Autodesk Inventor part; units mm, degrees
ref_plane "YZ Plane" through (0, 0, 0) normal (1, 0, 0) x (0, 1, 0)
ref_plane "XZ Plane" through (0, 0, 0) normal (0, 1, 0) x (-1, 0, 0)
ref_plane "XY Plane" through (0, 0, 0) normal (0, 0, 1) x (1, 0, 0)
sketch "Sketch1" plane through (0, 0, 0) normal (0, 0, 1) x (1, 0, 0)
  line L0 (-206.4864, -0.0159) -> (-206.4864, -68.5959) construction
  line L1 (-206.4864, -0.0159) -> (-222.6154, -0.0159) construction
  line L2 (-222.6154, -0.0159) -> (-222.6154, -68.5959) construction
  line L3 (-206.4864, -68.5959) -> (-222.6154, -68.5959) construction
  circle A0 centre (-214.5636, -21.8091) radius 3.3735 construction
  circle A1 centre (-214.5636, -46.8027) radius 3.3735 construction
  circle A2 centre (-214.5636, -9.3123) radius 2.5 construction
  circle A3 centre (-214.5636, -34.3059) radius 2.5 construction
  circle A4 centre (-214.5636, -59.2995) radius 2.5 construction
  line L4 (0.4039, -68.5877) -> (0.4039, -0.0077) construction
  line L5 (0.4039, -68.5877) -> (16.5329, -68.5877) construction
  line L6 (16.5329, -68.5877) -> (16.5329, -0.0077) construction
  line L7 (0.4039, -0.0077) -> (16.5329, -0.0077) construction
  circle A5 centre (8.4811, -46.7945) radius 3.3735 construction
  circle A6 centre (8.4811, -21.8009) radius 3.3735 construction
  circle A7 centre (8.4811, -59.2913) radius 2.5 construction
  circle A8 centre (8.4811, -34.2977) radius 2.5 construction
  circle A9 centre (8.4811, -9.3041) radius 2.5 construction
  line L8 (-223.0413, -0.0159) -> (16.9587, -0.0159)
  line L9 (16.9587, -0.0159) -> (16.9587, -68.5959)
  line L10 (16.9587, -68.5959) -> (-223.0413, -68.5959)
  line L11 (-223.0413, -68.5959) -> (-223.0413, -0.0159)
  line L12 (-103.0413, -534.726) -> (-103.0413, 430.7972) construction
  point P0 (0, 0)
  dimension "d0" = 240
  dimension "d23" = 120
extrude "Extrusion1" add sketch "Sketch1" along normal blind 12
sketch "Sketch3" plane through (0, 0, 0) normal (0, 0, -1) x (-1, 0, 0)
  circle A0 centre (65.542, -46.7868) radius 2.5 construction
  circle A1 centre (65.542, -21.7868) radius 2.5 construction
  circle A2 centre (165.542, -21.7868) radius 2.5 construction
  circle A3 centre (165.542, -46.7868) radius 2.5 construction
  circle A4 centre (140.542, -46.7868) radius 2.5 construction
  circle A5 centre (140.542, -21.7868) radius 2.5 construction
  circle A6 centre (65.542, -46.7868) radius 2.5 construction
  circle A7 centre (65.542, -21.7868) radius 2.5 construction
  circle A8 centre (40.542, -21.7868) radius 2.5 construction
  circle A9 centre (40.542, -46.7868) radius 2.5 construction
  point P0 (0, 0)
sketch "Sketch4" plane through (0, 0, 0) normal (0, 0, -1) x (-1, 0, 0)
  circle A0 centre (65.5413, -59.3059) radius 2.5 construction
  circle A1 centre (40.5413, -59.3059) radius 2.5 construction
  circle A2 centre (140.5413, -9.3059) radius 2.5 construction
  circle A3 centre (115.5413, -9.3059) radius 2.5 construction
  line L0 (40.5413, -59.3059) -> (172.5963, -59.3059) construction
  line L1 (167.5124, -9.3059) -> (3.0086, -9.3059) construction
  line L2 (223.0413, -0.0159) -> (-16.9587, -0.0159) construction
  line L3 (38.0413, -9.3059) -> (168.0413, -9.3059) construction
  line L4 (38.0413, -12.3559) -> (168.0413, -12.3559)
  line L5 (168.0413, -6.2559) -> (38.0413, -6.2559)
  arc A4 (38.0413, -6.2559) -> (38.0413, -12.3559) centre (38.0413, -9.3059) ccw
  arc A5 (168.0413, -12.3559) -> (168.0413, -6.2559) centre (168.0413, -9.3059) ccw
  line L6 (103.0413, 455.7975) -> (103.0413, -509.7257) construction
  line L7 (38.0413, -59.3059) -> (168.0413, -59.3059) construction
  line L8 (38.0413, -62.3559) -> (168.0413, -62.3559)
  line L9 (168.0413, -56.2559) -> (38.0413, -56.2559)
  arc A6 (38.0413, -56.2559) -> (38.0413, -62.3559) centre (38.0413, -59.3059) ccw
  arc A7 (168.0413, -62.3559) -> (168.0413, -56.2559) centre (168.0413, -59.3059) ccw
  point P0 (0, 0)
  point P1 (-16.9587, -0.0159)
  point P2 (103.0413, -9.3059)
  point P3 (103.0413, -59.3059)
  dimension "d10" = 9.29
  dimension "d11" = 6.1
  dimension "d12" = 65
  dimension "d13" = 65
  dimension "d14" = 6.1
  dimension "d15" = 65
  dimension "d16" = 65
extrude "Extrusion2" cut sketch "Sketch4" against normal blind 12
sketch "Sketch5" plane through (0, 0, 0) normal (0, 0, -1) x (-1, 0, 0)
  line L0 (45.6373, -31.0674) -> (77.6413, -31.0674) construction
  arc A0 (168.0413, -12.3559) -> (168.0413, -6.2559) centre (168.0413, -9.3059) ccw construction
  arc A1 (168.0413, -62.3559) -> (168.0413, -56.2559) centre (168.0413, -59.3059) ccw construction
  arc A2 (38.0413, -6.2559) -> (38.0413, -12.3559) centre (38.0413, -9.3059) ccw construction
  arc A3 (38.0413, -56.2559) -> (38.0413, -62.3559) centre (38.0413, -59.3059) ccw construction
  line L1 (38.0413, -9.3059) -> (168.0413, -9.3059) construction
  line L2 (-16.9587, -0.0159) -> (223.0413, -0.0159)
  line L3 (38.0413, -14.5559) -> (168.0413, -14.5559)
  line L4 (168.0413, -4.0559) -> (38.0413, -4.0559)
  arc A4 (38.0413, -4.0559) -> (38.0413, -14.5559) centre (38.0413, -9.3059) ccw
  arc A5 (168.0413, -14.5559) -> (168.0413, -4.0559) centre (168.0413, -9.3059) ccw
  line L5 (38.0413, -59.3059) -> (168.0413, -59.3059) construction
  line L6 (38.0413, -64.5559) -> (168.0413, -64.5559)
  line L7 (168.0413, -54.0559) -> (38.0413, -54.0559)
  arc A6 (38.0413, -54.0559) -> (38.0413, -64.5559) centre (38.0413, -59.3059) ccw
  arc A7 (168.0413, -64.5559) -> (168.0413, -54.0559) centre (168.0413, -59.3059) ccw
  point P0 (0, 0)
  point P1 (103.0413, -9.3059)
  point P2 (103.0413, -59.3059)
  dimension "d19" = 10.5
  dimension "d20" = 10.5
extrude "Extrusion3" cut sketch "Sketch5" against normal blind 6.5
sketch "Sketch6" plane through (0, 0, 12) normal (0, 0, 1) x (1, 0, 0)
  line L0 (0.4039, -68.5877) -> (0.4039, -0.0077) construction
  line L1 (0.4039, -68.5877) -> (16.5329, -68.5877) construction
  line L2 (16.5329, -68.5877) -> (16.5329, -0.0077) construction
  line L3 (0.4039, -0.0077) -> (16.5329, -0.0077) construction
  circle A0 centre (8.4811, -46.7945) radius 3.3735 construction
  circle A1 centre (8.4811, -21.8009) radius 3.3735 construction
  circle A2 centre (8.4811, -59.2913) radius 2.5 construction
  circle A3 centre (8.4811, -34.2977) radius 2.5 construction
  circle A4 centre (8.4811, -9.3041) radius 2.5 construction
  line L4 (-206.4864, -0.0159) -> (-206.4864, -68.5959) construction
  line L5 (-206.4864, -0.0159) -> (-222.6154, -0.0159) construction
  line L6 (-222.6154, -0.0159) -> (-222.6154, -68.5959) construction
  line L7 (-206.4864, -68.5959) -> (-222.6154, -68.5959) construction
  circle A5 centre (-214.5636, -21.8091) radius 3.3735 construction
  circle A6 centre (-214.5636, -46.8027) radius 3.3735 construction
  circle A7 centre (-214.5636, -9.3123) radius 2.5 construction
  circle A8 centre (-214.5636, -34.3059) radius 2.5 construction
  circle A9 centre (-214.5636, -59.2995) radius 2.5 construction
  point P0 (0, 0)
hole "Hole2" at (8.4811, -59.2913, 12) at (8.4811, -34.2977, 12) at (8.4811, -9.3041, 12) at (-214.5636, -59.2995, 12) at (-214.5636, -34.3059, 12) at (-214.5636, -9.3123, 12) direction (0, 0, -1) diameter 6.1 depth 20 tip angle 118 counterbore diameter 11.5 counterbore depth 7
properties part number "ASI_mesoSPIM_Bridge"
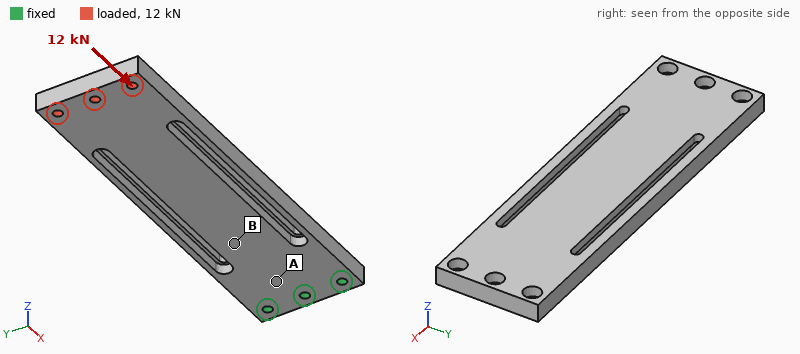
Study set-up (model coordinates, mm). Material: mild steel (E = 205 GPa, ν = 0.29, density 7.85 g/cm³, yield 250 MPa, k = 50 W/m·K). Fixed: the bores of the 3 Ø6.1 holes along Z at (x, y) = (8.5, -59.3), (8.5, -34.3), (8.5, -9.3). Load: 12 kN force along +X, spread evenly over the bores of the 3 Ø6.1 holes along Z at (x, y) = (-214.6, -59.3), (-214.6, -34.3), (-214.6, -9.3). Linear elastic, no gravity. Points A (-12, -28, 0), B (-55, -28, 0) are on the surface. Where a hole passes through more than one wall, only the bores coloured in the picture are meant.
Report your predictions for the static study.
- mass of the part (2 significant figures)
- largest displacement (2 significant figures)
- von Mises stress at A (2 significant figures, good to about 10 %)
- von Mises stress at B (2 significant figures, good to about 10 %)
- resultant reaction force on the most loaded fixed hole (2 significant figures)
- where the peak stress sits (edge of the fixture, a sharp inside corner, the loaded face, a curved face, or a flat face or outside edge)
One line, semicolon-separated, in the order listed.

1.3 kg; 0.69 mm; 41 MPa; 56 MPa; 4.3 kN; the loaded face
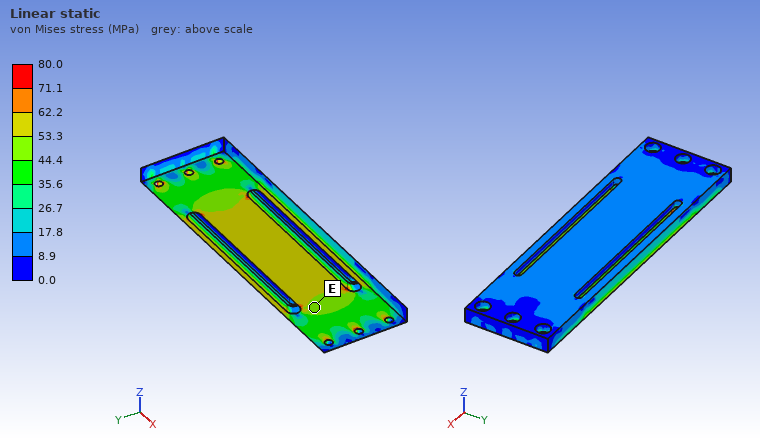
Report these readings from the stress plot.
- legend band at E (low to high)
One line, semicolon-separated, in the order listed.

44.4 to 53.3 MPa
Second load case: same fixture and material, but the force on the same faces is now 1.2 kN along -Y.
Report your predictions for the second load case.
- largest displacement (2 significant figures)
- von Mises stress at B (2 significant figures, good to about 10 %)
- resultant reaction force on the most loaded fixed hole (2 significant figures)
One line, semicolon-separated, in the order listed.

0.15 mm; 14 MPa; 5.1 kN
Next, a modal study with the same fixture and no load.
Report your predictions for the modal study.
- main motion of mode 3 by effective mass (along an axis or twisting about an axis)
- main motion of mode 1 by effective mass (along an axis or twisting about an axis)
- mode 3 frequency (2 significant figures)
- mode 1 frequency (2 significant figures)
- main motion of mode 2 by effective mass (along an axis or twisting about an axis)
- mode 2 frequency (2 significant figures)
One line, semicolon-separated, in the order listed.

along Z; along Z; 1000 Hz; 160 Hz; along Y; 760 Hz
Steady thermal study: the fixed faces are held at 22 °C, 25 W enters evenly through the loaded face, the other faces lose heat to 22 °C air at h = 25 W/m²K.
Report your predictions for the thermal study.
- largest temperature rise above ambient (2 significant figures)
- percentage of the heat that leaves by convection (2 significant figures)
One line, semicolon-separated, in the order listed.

60 K; 87 %
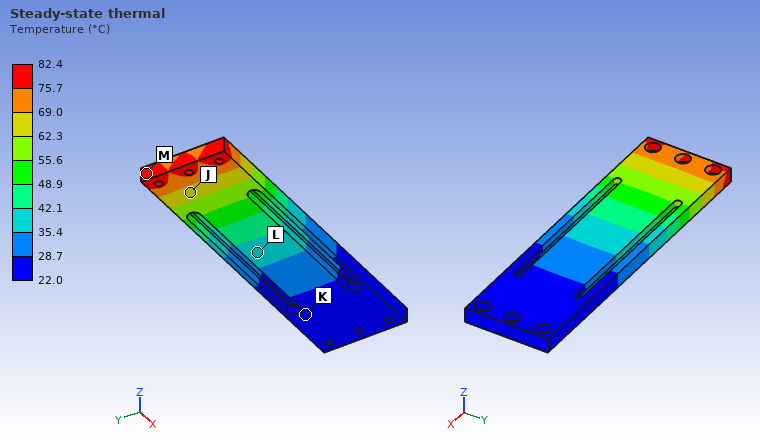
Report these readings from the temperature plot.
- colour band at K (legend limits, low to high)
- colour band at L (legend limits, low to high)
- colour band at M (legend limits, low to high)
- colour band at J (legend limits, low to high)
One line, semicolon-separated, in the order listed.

22.0 to 28.7 °C; 35.4 to 42.1 °C; 75.7 to 82.4 °C; 62.3 to 69.0 °C
